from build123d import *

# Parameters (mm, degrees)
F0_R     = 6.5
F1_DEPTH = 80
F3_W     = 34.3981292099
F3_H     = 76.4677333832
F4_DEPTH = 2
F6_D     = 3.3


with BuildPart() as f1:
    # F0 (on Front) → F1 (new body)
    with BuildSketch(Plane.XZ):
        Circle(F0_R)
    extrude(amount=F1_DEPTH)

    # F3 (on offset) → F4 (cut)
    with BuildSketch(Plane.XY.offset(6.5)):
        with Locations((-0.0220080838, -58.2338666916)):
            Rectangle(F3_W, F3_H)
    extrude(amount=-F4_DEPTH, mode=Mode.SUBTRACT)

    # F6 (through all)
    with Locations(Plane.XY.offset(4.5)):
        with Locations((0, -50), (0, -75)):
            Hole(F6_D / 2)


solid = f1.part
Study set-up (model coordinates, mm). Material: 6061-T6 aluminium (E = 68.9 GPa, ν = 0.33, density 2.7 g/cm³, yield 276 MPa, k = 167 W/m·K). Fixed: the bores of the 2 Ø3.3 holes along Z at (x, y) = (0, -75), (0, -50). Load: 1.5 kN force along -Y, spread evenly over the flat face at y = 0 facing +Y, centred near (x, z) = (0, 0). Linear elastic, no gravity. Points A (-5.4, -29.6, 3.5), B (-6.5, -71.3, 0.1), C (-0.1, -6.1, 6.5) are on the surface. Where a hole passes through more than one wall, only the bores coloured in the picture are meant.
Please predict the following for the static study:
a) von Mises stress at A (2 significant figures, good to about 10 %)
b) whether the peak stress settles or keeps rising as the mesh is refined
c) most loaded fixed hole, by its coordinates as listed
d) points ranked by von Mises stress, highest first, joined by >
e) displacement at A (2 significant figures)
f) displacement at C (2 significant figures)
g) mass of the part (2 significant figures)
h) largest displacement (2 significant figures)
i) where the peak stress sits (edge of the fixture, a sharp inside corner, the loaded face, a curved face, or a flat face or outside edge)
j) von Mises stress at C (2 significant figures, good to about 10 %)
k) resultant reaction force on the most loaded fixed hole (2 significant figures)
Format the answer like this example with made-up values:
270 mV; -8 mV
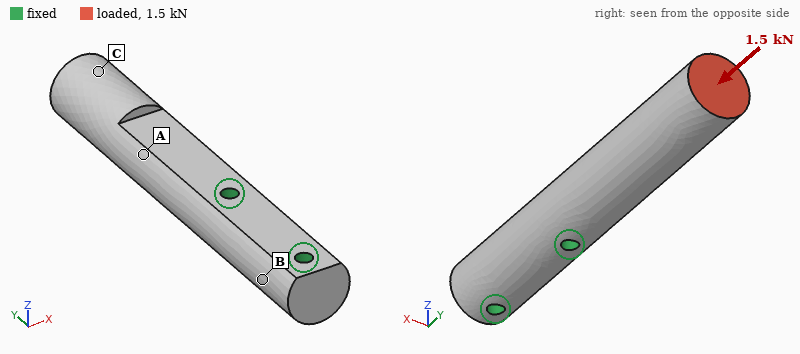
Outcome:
16 MPa; keeps rising; (0, -50); A > C > B; 6.0 µm; 17 µm; 26 g; 19 µm; edge of the fixture; 11 MPa; 1.4 kN
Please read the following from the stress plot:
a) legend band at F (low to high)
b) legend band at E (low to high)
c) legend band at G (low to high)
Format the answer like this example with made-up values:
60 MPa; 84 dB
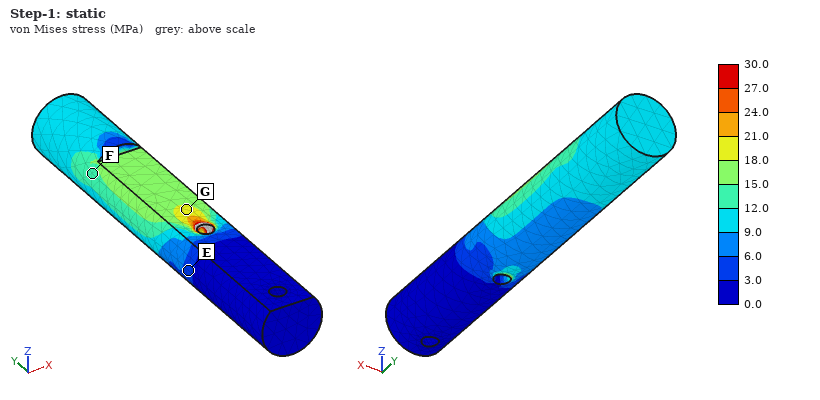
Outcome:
12.0 to 15.0 MPa; 3.0 to 6.0 MPa; 18.0 to 21.0 MPa
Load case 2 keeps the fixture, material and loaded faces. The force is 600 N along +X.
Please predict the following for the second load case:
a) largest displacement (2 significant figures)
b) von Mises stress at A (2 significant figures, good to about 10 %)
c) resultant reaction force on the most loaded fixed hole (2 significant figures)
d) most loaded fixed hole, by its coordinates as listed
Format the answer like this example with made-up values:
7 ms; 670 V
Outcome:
0.35 mm; 72 MPa; 1.3 kN; (0, -50)
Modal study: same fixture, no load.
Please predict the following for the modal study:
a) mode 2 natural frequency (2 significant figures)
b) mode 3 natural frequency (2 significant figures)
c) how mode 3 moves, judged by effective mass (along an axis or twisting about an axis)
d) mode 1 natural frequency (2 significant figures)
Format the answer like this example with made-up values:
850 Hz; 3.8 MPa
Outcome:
3100 Hz; 14 kHz; twisting about Y; 3000 Hz
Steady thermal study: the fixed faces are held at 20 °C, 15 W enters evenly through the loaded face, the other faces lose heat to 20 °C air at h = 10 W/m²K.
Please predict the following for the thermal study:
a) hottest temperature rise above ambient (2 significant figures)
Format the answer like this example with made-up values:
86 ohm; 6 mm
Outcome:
35 K
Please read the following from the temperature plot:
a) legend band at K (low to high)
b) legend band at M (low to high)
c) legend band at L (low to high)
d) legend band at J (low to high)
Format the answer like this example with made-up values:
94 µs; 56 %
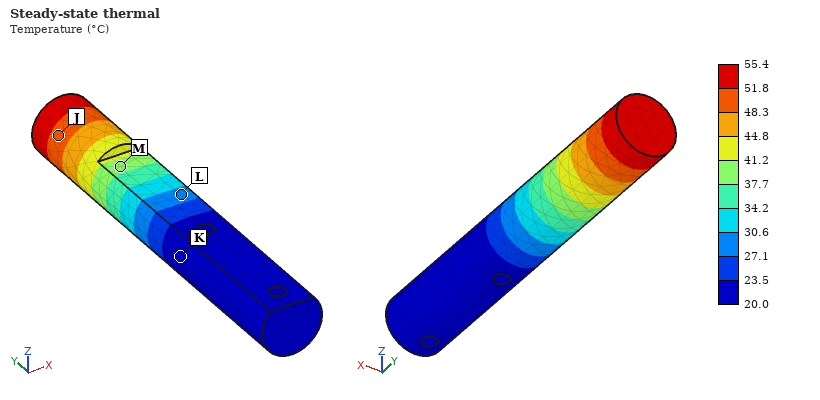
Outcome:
20.0 to 23.5 °C; 37.7 to 41.2 °C; 27.1 to 30.6 °C; 48.3 to 51.8 °C
